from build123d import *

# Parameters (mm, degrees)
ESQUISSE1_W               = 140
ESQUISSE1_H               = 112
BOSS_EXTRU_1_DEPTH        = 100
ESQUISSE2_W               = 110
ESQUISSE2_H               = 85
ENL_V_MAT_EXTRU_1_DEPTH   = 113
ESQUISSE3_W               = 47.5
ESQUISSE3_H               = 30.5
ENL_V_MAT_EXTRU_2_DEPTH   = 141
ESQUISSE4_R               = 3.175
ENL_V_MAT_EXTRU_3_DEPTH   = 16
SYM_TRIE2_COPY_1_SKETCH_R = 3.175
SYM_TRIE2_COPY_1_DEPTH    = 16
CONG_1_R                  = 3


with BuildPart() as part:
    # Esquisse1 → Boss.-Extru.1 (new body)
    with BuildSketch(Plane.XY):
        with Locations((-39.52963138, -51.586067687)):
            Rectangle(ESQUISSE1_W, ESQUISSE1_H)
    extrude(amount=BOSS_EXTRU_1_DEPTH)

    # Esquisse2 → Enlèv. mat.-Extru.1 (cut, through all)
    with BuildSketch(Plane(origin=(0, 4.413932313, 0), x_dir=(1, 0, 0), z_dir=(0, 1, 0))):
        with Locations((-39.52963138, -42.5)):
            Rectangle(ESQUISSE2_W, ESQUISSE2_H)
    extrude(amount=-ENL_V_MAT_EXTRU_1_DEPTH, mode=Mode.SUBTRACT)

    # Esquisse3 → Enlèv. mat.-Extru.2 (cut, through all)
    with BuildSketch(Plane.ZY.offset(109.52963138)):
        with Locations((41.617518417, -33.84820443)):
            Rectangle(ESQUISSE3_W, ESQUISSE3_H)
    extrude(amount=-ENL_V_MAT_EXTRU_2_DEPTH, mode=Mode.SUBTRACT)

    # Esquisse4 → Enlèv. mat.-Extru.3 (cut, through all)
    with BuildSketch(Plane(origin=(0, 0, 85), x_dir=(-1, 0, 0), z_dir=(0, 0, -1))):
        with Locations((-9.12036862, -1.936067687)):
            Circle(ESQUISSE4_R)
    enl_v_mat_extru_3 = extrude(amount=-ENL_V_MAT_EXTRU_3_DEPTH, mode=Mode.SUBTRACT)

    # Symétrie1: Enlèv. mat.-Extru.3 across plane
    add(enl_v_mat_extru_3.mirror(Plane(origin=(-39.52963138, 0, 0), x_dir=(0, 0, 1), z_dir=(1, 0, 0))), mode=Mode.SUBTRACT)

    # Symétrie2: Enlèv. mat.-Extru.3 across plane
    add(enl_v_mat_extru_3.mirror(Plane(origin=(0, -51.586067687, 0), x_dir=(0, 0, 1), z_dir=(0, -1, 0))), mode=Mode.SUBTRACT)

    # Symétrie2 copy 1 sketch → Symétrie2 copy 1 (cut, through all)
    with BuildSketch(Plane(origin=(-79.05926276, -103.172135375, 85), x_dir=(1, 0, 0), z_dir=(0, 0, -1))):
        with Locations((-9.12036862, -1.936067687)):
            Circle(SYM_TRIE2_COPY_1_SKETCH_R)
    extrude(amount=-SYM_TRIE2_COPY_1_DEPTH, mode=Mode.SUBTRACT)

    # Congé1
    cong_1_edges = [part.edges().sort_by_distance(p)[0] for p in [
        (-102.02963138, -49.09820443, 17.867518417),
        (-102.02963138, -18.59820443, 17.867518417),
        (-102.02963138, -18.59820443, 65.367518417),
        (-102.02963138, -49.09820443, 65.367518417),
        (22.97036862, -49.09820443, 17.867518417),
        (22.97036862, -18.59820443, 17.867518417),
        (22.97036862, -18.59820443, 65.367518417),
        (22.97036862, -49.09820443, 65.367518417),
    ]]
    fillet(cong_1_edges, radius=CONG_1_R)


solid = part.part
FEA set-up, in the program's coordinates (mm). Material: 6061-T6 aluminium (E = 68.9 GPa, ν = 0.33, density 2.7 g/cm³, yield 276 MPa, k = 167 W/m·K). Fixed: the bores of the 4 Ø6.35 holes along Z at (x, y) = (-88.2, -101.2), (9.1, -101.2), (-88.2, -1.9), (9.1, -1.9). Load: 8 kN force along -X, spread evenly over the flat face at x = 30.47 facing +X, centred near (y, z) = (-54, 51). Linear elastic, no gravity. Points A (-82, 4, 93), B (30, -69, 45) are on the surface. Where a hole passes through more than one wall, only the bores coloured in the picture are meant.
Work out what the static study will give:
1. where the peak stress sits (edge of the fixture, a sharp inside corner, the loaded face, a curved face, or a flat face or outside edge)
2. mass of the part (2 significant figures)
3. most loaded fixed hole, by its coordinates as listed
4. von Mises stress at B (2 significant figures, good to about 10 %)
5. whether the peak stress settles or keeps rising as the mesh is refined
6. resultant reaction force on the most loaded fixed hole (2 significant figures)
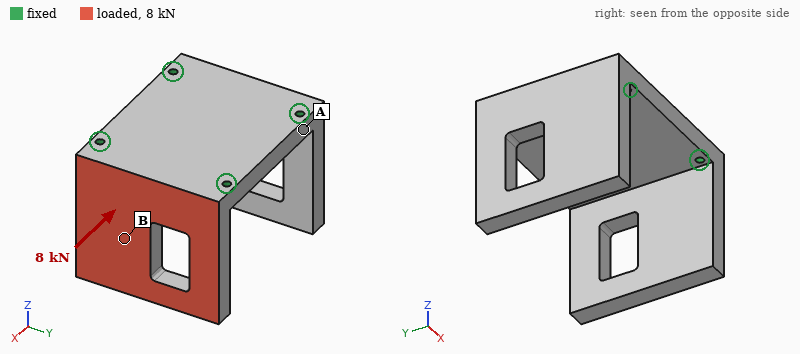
edge of the fixture
1.3 kg
(9.1, -101.2)
25 MPa
keeps rising
3.0 kN
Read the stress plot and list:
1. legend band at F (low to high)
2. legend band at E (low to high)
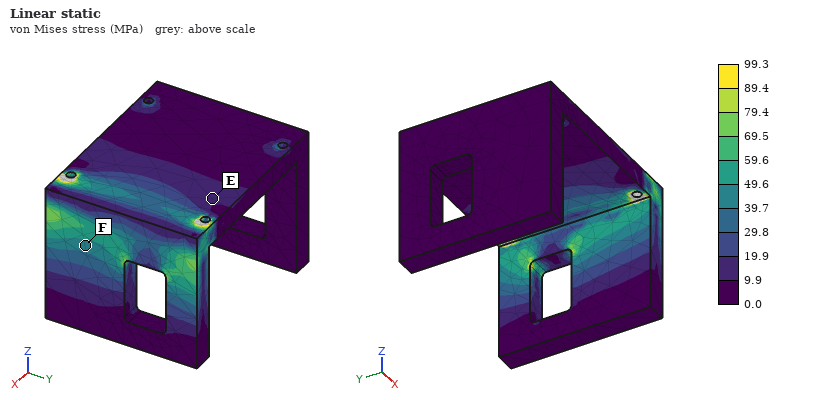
39.7 to 49.6 MPa
9.9 to 19.9 MPa
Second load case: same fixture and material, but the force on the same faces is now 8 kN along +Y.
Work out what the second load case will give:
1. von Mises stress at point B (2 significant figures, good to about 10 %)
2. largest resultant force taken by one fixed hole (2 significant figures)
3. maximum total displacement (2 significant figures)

13 MPa
5.5 kN
56 µm
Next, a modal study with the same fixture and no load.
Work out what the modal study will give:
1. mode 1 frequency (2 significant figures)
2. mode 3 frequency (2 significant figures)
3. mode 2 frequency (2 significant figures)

1100 Hz
2400 Hz
1100 Hz
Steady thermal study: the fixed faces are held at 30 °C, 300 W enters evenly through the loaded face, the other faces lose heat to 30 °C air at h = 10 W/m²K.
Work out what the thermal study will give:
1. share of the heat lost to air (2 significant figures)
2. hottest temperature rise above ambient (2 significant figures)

4.1 %
78 K
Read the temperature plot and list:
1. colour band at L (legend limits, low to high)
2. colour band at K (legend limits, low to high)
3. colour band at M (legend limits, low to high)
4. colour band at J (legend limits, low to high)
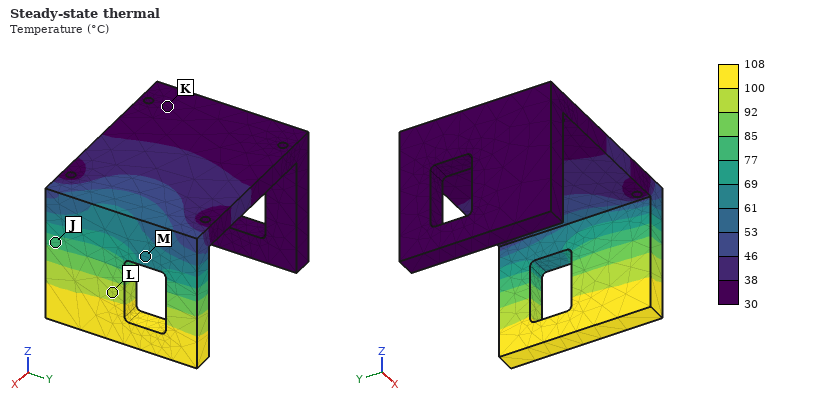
92 to 100 °C
30 to 38 °C
61 to 69 °C
77 to 85 °C
